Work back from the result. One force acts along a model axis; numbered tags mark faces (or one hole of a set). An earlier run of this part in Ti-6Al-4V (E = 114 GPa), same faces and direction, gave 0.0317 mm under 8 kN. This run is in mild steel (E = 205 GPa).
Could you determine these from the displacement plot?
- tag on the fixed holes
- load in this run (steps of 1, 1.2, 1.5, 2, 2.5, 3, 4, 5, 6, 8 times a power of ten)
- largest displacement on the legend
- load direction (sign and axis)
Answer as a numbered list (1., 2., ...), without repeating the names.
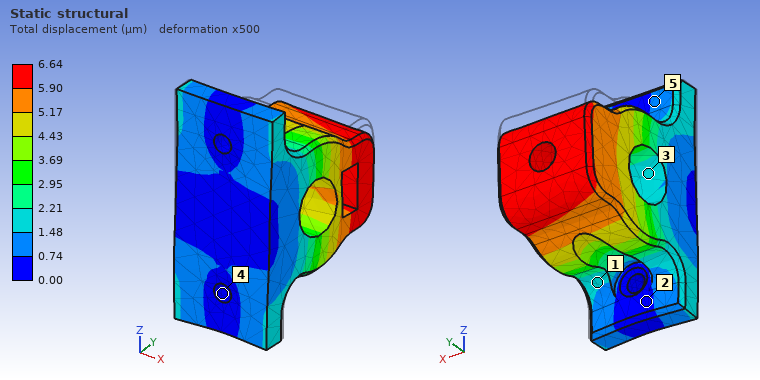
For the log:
1. 4
2. 3 kN
3. 6.64 µm
4. -Z
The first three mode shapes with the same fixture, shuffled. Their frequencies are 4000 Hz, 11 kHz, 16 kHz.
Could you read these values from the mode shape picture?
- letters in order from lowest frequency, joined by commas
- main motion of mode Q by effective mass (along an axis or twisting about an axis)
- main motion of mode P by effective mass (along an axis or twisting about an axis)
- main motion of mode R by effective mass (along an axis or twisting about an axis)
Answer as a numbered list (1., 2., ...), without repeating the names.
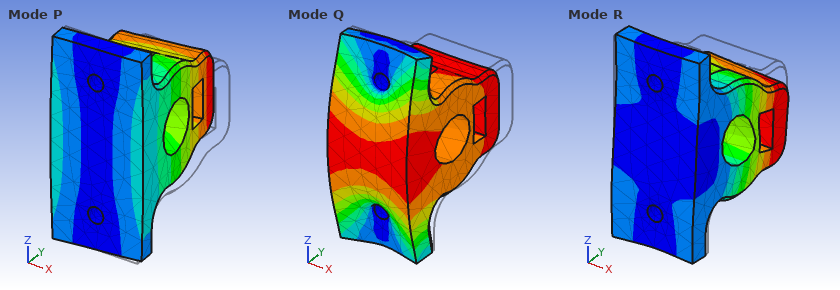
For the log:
1. P, R, Q
2. along Y
3. along X
4. along Z
